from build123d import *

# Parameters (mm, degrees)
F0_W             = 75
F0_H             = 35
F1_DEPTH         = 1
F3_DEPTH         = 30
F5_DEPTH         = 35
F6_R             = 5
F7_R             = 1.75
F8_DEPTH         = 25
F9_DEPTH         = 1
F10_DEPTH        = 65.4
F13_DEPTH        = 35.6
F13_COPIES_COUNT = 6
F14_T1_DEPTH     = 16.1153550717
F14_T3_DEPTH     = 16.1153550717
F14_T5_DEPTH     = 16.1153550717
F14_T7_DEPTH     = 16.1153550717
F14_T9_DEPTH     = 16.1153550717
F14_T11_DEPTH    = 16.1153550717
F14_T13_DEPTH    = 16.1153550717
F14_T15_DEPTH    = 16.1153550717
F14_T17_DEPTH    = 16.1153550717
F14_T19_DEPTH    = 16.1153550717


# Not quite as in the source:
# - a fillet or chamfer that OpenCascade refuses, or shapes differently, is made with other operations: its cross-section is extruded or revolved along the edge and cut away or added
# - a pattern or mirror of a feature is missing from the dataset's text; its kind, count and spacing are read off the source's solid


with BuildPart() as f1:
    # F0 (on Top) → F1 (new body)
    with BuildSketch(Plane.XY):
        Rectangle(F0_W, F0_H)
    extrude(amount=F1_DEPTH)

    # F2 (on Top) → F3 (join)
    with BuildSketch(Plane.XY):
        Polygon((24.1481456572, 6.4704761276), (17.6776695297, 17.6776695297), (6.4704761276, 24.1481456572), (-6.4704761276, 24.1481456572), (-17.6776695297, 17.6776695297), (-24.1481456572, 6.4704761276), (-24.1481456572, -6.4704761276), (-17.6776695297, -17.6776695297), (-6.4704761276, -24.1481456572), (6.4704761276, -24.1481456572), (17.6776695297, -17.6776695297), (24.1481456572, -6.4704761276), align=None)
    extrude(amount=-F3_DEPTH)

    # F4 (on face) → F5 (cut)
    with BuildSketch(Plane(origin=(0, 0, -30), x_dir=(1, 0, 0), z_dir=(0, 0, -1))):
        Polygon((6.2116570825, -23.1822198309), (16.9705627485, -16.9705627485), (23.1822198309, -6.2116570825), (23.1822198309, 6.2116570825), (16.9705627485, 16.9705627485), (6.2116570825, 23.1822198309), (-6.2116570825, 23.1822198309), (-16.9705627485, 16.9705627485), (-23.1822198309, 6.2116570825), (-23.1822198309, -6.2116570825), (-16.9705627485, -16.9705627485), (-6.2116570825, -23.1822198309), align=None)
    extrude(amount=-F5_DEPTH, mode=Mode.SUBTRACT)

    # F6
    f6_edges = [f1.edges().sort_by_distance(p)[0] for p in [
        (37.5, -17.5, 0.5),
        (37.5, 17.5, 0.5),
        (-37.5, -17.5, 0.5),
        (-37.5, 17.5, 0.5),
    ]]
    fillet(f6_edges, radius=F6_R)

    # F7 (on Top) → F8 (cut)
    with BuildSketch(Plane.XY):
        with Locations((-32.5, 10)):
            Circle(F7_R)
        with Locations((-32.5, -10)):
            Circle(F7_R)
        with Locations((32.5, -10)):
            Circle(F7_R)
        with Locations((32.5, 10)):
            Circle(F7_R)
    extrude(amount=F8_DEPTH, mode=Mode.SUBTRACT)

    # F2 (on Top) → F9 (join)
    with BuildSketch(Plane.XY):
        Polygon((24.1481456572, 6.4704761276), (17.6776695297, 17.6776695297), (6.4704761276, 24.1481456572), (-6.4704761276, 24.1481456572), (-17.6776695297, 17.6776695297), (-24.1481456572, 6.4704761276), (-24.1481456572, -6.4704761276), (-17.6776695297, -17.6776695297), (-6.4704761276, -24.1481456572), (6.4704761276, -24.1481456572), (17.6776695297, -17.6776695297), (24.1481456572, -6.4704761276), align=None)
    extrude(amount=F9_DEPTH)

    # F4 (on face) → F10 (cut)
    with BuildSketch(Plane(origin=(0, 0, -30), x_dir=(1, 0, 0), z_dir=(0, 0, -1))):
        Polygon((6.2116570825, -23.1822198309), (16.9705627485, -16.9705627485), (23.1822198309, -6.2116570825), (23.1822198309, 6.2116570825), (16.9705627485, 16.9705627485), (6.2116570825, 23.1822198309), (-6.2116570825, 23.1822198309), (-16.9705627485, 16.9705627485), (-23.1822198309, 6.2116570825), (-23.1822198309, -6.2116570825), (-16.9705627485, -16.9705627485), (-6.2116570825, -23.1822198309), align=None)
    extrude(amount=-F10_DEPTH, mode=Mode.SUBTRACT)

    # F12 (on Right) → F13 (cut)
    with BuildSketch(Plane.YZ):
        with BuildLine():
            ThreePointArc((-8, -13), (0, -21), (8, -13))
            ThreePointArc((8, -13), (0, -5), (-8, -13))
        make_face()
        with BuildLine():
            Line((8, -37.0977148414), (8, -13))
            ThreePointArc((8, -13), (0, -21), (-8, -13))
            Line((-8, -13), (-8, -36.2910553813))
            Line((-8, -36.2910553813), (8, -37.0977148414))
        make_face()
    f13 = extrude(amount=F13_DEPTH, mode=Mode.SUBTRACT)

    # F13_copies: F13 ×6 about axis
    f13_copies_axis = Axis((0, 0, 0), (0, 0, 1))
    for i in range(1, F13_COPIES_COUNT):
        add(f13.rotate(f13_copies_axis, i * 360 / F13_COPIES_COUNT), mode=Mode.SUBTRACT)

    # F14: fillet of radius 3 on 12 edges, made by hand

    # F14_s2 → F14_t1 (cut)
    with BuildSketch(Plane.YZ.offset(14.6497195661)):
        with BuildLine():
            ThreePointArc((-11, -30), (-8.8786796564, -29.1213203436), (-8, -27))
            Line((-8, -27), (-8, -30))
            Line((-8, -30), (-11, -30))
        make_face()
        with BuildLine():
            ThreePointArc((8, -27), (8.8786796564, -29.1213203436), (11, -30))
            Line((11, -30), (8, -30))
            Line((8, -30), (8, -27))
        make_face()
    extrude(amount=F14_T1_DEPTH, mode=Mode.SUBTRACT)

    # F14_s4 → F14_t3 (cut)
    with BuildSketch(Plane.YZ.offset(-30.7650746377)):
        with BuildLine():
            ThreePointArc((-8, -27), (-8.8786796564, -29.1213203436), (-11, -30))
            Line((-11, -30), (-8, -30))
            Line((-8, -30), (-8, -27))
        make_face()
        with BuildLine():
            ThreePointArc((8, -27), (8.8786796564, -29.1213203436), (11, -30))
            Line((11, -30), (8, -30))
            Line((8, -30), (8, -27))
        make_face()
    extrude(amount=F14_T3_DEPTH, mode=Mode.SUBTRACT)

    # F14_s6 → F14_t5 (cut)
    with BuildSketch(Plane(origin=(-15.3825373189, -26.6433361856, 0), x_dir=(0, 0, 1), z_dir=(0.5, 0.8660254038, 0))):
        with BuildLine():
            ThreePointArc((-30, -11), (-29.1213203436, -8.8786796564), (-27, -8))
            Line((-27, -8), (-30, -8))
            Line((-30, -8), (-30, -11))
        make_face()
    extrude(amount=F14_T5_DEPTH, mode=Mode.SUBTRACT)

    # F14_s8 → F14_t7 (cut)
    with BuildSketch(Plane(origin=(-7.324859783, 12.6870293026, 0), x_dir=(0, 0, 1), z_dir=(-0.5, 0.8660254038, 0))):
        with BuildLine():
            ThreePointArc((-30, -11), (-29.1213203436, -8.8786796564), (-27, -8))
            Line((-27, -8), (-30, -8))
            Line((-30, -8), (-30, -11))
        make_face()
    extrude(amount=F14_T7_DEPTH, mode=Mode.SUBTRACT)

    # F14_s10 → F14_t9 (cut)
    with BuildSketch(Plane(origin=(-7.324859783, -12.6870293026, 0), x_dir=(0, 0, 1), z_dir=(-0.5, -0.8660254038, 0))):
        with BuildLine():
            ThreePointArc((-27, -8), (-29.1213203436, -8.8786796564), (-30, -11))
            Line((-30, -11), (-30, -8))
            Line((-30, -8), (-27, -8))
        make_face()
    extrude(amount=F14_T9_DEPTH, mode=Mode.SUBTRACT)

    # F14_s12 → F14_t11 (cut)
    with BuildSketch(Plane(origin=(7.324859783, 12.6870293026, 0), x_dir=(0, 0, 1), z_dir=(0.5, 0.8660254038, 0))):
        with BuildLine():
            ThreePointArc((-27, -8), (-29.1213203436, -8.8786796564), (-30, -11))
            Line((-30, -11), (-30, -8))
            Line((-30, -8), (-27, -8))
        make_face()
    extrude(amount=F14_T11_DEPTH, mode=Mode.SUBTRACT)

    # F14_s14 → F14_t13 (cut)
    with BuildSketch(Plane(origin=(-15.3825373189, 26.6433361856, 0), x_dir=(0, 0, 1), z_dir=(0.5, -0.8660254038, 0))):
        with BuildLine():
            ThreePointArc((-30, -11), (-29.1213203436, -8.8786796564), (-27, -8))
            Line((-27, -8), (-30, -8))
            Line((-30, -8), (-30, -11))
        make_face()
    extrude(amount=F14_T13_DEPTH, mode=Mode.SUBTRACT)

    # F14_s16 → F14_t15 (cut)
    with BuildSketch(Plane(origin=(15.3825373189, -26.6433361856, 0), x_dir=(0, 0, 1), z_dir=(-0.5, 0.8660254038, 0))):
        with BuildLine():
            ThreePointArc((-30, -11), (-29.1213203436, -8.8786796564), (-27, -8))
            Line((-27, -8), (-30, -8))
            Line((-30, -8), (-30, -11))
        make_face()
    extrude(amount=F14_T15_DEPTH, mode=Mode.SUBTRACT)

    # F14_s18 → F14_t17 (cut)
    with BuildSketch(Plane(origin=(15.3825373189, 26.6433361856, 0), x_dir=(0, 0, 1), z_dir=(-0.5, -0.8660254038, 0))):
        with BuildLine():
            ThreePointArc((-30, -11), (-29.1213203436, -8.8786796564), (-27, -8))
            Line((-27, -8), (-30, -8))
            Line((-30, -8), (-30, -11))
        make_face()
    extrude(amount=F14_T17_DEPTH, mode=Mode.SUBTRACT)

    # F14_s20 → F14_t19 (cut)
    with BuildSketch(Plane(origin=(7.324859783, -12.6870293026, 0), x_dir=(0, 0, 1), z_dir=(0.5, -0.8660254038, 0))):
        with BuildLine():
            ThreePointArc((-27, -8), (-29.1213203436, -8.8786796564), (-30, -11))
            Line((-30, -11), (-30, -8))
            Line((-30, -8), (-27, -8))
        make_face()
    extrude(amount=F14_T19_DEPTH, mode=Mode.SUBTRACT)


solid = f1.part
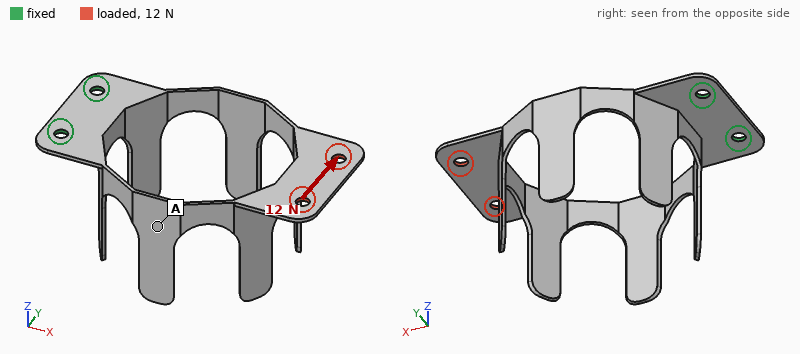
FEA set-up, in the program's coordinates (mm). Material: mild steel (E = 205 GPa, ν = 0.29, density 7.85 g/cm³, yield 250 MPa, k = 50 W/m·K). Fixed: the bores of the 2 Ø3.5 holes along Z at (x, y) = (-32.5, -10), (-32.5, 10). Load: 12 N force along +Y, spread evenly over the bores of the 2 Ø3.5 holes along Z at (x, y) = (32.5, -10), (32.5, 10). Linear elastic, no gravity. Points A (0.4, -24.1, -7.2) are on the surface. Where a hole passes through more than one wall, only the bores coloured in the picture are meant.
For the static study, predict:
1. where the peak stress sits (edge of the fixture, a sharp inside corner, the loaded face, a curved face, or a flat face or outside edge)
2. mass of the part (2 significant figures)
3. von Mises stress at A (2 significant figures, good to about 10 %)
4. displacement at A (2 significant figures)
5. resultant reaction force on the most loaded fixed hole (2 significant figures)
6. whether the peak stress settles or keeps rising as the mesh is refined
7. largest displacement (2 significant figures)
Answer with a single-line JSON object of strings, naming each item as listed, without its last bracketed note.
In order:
{"where the peak stress sits": "a sharp inside corner", "mass of the part": "26 g", "von Mises stress at A": "14 MPa", "displacement at A": "0.19 mm", "resultant reaction force on the most loaded fixed hole": "32 N", "whether the peak stress settles or keeps rising as the mesh is refined": "keeps rising", "largest displacement": "0.34 mm"}
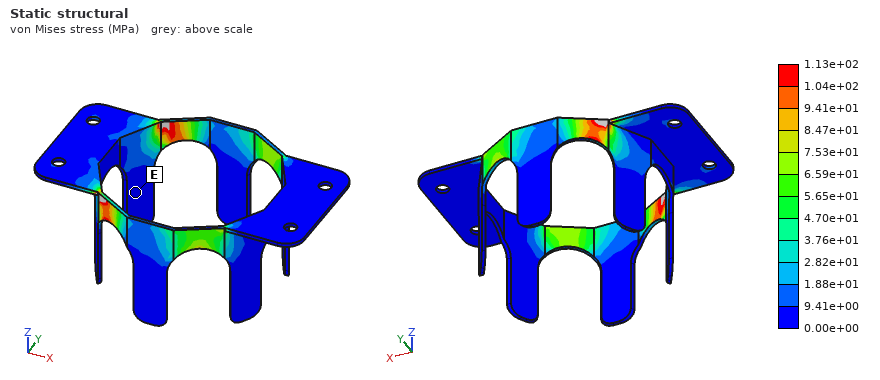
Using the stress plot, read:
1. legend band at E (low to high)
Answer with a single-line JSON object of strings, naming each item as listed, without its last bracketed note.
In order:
{"legend band at E": "0.00e+00 to 9.41e+00 MPa"}
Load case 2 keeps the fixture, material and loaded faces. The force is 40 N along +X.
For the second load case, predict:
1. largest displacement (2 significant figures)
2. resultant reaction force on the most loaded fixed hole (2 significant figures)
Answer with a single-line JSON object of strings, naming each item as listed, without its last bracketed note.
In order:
{"largest displacement": "79 µm", "resultant reaction force on the most loaded fixed hole": "25 N"}
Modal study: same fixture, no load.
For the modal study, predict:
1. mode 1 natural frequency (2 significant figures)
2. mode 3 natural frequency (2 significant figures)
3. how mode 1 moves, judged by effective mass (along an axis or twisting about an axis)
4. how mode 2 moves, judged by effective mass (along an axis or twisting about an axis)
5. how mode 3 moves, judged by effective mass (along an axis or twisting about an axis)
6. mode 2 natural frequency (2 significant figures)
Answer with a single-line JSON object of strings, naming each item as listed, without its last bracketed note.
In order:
{"mode 1 natural frequency": "160 Hz", "mode 3 natural frequency": "490 Hz", "how mode 1 moves, judged by effective mass": "along Z", "how mode 2 moves, judged by effective mass": "along Y", "how mode 3 moves, judged by effective mass": "twisting about X", "mode 2 natural frequency": "280 Hz"}
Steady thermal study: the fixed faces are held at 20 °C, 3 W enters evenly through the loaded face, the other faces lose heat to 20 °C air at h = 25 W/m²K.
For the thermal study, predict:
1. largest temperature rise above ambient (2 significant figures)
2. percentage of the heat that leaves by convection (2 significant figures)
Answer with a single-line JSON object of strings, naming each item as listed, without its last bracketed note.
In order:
{"largest temperature rise above ambient": "54 K", "percentage of the heat that leaves by convection": "95 %"}
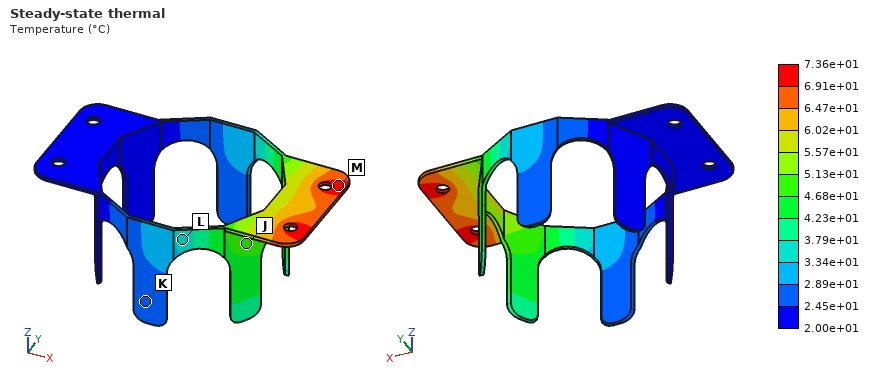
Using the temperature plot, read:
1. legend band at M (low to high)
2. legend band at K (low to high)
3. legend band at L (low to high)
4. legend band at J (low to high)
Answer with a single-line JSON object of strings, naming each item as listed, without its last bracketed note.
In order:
{"legend band at M": "6.91e+01 to 7.36e+01 °C", "legend band at K": "2.45e+01 to 2.89e+01 °C", "legend band at L": "3.34e+01 to 3.79e+01 °C", "legend band at J": "4.68e+01 to 5.13e+01 °C"}
